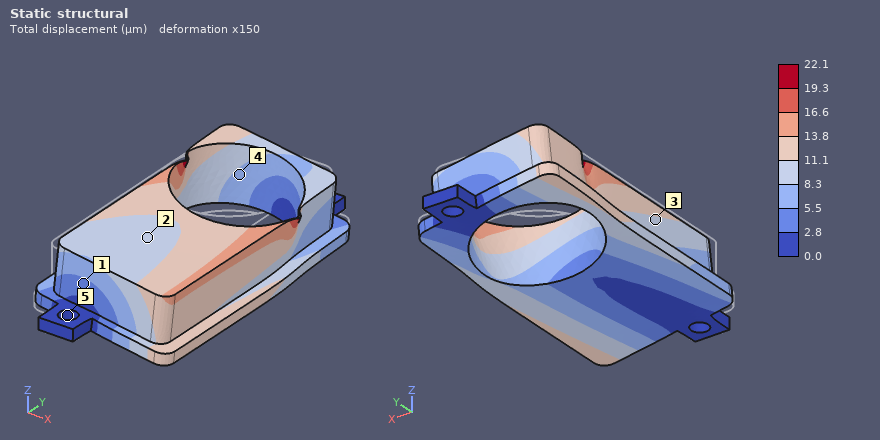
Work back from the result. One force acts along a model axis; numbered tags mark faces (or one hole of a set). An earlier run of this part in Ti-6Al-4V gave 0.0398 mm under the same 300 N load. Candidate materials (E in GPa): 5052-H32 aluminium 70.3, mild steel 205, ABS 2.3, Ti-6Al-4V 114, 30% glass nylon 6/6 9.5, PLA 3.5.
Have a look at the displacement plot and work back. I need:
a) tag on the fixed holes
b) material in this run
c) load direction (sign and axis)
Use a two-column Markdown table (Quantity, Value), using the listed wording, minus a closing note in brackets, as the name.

| Quantity | Value |
|---|---|
| tag on the fixed holes | 5 |
| material in this run | mild steel |
| load direction | +X |
